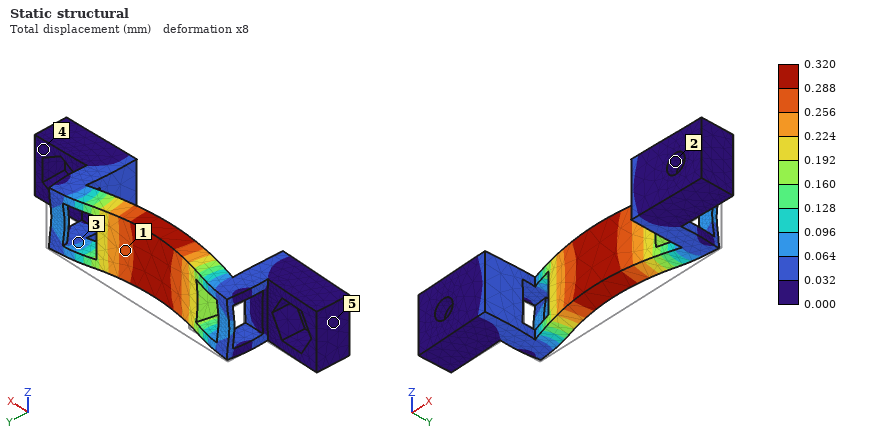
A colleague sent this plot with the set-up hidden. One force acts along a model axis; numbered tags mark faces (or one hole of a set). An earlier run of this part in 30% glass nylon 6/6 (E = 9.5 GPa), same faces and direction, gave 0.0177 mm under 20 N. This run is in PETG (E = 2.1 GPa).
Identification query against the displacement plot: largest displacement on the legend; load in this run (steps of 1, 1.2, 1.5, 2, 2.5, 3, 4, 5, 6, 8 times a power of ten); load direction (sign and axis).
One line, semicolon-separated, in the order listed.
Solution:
0.320 mm; 80 N; -Y
